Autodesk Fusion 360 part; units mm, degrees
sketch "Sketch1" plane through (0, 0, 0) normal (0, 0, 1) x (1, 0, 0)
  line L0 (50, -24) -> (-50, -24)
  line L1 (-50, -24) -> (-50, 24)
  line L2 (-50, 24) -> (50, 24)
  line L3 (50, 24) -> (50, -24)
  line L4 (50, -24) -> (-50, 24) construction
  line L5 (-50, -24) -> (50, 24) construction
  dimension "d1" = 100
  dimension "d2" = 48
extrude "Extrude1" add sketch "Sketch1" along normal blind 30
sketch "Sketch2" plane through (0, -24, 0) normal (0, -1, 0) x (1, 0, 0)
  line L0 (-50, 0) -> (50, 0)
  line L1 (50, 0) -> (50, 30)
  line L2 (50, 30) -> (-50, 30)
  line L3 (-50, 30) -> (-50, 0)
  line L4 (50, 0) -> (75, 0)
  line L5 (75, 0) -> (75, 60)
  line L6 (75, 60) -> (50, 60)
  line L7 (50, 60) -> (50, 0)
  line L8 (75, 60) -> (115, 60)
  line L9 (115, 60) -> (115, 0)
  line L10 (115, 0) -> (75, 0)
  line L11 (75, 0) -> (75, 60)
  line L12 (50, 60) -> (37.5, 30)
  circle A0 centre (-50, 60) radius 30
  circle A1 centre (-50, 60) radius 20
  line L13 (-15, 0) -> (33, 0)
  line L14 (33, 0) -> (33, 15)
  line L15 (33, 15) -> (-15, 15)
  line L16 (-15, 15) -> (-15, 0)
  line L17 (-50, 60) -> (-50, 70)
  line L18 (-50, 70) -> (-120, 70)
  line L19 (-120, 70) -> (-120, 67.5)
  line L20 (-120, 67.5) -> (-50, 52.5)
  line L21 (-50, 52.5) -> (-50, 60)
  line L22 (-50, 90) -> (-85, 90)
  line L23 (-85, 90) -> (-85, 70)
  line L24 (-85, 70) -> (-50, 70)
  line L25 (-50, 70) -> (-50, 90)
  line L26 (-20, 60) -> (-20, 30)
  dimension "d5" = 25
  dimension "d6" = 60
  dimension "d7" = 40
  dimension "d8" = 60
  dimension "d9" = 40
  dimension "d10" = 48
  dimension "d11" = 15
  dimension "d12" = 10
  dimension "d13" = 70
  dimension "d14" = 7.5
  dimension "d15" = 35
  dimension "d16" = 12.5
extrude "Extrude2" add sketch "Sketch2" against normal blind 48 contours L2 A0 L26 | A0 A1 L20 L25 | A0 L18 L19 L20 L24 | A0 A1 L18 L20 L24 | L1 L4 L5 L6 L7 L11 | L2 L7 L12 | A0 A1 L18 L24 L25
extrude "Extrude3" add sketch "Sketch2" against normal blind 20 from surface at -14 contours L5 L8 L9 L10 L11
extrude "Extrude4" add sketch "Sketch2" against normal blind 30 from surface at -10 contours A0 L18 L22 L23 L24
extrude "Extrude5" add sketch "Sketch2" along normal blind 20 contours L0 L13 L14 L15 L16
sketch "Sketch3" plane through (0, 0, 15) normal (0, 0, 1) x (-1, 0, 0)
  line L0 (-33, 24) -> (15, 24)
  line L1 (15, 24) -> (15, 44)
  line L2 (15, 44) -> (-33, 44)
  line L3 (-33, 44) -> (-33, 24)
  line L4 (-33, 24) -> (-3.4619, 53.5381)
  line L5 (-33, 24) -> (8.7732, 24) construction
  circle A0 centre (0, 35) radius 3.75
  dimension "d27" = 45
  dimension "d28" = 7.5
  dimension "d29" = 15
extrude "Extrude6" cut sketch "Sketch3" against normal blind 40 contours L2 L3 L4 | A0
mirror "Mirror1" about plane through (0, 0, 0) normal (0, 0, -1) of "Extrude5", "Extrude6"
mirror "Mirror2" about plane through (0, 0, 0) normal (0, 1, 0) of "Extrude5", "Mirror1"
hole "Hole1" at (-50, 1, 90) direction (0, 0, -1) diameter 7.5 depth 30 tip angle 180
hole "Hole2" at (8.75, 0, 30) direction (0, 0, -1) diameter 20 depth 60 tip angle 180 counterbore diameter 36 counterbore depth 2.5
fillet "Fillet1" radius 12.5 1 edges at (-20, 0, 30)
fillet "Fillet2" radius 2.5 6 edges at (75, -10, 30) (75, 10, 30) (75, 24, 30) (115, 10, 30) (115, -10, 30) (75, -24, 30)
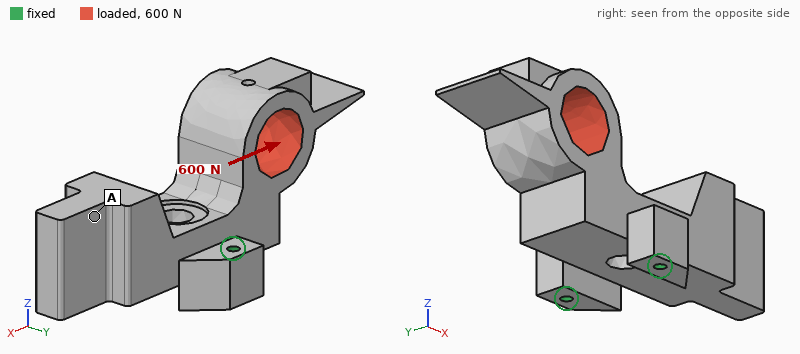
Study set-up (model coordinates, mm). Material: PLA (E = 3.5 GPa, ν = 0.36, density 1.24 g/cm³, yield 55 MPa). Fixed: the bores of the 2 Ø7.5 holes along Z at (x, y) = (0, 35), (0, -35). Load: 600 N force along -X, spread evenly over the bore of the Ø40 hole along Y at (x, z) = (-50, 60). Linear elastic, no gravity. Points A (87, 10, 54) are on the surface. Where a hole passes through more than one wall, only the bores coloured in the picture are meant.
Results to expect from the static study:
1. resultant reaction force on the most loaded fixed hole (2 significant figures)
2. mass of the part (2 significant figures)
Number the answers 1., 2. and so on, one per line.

1. 330 N
2. 510 g
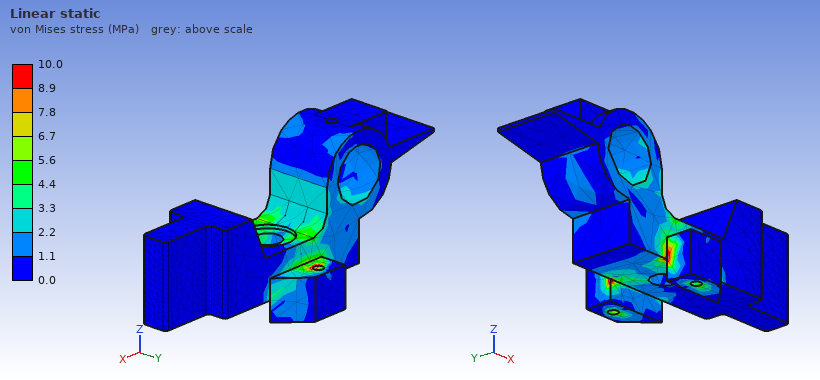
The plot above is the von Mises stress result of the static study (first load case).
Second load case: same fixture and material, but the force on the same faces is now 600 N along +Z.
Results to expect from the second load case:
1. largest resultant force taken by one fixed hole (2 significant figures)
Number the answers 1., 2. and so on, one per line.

1. 410 N
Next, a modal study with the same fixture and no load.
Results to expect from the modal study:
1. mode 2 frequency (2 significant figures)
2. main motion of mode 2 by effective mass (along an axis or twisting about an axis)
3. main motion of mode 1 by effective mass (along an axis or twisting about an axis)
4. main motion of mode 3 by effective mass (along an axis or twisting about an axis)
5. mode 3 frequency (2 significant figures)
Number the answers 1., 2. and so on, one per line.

1. 540 Hz
2. along Z
3. along X
4. along Y
5. 720 Hz
